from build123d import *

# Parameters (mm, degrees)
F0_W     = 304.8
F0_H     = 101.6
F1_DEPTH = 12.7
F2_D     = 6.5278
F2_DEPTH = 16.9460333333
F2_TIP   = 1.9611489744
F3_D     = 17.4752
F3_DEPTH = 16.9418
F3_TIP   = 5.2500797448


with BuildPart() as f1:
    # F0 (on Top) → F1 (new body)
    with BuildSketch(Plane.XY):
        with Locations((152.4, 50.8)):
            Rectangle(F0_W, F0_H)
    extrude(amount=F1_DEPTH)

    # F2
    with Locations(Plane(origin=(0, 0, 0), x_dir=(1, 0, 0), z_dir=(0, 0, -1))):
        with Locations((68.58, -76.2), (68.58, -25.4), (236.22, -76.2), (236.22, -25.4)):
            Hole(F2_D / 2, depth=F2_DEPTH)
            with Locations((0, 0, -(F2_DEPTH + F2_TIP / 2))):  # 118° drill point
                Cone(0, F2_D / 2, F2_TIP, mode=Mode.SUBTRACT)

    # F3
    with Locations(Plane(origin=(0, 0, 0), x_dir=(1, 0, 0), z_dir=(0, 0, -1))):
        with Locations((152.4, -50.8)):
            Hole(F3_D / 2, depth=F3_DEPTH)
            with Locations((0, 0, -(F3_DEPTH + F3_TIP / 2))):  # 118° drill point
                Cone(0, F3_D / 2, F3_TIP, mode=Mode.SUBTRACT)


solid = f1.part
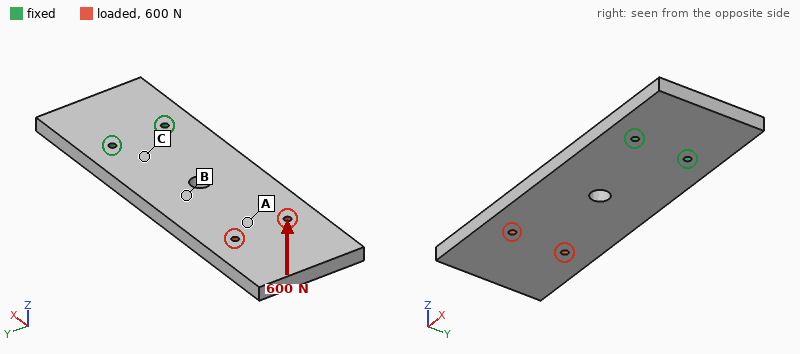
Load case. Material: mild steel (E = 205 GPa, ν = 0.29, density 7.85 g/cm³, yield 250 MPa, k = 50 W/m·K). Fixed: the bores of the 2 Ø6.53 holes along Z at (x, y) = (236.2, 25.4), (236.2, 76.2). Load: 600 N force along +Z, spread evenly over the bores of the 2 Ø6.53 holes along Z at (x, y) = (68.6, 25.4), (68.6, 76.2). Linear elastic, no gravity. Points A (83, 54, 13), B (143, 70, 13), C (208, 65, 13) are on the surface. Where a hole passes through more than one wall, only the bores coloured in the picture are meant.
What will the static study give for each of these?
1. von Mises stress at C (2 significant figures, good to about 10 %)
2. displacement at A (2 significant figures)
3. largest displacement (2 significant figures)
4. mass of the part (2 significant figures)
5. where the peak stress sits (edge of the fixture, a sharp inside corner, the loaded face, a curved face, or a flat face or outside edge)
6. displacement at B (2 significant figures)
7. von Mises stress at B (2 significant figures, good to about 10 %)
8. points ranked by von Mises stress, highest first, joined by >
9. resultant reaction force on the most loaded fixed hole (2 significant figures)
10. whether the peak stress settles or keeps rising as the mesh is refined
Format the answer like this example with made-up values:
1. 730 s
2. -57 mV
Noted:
1. 28 MPa
2. 0.26 mm
3. 0.47 mm
4. 3.1 kg
5. edge of the fixture
6. 0.11 mm
7. 19 MPa
8. C > B > A
9. 300 N
10. keeps rising
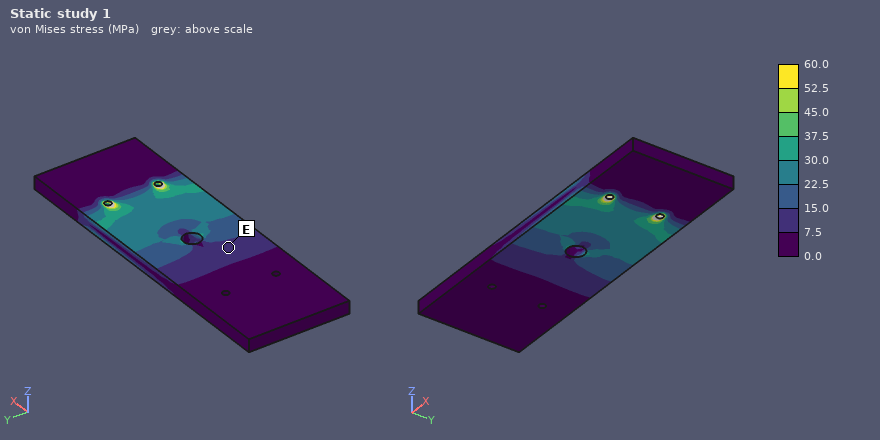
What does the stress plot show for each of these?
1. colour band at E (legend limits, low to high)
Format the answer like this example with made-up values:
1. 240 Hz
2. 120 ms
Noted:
1. 7.5 to 15.0 MPa
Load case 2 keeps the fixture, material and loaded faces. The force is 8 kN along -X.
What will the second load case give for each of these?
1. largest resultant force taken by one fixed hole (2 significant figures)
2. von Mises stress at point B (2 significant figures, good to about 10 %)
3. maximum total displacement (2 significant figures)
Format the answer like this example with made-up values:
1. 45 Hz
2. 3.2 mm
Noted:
1. 4.0 kN
2. 7.6 MPa
3. 6.5 µm
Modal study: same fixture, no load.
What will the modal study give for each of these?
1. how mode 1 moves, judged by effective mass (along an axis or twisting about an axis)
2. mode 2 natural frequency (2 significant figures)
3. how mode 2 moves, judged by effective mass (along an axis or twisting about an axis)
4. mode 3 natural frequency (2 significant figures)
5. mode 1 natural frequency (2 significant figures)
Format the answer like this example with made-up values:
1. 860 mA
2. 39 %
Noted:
1. along Z
2. 860 Hz
3. twisting about X
4. 1100 Hz
5. 180 Hz
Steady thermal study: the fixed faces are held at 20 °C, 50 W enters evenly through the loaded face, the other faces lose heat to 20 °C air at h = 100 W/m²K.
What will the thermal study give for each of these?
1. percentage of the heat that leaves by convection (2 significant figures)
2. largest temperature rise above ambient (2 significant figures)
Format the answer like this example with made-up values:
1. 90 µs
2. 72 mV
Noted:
1. 97 %
2. 28 K
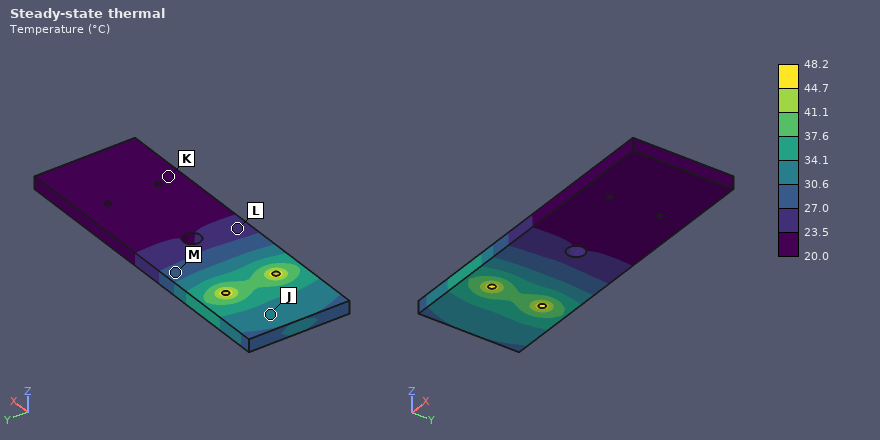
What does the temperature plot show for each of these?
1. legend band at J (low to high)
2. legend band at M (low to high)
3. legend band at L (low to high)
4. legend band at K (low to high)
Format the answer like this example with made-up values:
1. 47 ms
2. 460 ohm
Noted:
1. 30.6 to 34.1 °C
2. 27.0 to 30.6 °C
3. 23.5 to 27.0 °C
4. 20.0 to 23.5 °C
